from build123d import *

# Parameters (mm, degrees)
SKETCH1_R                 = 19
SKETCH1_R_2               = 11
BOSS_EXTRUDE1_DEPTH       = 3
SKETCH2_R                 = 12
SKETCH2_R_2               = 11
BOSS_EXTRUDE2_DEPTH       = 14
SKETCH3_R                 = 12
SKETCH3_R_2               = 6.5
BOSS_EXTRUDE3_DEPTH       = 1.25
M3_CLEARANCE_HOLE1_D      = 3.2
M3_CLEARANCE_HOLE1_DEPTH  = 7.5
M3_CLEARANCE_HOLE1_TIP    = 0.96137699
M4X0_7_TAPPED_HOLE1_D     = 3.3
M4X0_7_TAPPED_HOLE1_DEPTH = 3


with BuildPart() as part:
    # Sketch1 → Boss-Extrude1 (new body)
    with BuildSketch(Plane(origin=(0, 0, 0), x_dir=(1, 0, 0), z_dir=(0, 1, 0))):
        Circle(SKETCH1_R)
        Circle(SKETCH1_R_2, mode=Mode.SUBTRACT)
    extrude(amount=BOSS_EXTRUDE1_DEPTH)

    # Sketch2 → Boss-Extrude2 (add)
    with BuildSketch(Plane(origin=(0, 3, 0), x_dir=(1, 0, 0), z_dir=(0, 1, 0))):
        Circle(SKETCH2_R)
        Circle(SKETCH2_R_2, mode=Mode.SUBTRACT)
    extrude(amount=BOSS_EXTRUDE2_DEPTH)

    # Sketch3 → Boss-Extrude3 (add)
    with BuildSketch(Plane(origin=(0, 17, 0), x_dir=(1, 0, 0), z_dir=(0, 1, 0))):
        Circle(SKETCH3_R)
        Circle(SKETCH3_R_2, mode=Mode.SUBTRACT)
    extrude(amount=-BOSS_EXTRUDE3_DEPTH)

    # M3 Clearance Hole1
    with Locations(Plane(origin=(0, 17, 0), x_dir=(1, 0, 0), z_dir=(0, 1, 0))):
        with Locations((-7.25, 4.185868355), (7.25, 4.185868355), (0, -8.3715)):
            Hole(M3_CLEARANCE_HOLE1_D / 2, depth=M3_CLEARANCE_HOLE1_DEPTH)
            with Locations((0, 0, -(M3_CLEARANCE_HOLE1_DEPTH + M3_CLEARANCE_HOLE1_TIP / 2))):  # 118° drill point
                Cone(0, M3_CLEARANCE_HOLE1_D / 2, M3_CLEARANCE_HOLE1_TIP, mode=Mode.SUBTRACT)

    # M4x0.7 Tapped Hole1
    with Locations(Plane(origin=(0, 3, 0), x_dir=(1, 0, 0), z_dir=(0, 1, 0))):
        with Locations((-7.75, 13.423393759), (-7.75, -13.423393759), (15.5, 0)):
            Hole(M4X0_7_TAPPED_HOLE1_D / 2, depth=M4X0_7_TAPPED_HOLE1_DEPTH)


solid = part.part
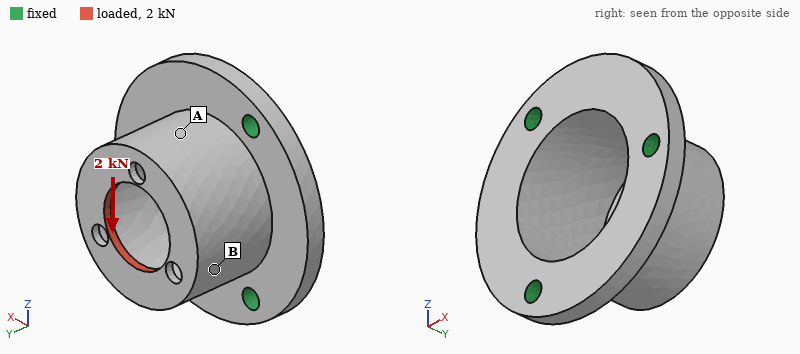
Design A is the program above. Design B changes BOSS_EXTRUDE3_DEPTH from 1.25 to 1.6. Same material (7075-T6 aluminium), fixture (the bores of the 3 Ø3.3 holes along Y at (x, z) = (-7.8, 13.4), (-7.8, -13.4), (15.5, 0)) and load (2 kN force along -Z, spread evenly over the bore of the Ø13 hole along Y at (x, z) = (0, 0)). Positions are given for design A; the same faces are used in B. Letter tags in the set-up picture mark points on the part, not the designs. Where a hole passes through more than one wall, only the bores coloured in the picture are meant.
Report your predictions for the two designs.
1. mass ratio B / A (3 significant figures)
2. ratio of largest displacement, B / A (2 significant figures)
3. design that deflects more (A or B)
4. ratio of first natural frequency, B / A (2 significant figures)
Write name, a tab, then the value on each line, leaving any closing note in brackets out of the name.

mass ratio B / A	1.02
ratio of largest displacement, B / A	0.90
design that deflects more	A
ratio of first natural frequency, B / A	0.99
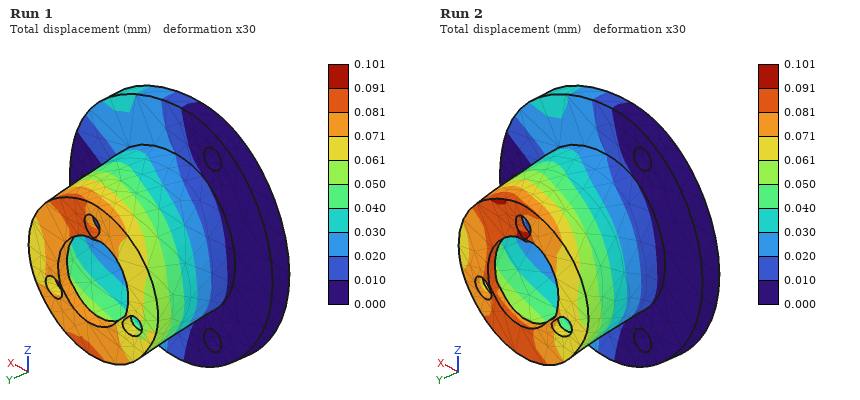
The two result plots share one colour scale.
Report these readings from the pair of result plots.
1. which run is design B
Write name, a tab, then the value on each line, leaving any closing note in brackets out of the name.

which run is design B	Run 1
